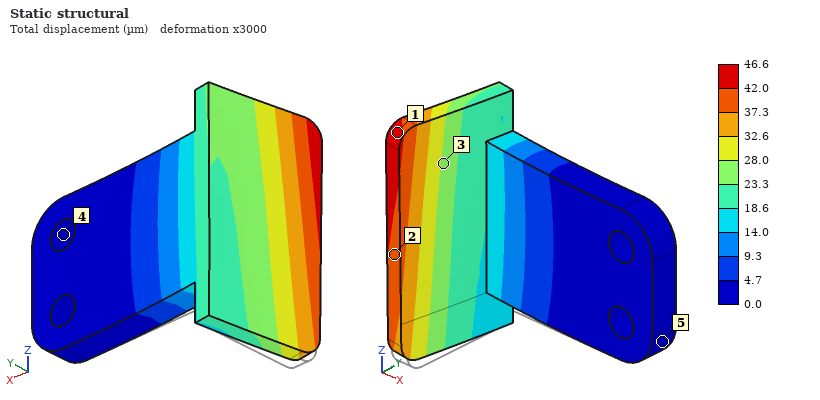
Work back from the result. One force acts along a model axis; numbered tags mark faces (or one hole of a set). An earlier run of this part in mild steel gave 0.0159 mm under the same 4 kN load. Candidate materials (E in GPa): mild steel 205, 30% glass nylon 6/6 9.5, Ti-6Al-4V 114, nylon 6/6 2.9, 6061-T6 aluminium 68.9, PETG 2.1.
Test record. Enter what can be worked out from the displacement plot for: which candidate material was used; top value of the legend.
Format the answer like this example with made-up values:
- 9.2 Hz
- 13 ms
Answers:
- 6061-T6 aluminium
- 46.6 µm
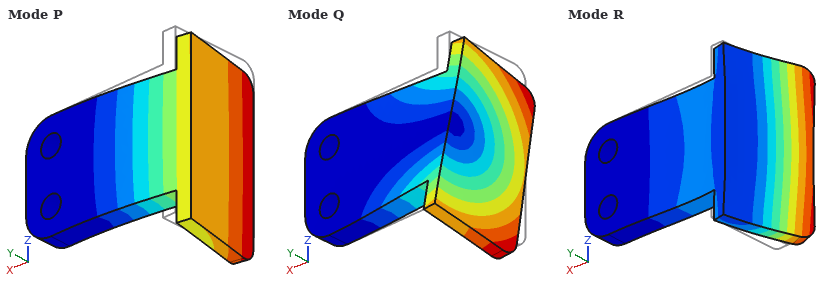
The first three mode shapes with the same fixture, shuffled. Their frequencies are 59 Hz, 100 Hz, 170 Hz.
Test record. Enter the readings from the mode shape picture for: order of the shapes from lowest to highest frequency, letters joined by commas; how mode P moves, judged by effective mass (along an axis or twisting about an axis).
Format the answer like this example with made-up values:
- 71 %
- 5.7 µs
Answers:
- P, Q, R
- along Y
